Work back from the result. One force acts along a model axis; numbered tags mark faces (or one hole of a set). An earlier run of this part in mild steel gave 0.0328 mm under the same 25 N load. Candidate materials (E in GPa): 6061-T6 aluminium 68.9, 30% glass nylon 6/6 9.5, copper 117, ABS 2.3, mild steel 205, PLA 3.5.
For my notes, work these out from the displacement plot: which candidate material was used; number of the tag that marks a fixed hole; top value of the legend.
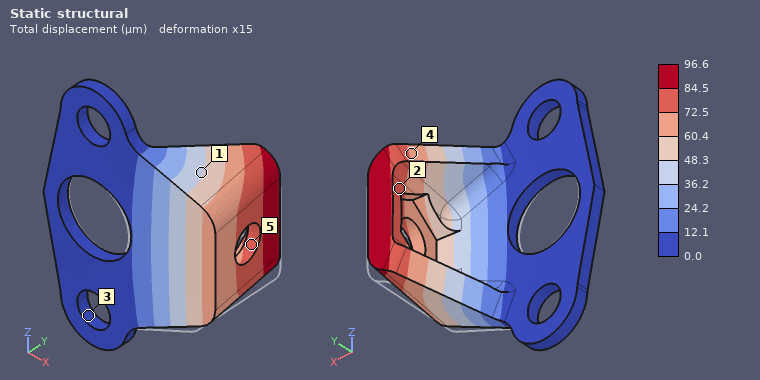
6061-T6 aluminium
3
96.6 µm
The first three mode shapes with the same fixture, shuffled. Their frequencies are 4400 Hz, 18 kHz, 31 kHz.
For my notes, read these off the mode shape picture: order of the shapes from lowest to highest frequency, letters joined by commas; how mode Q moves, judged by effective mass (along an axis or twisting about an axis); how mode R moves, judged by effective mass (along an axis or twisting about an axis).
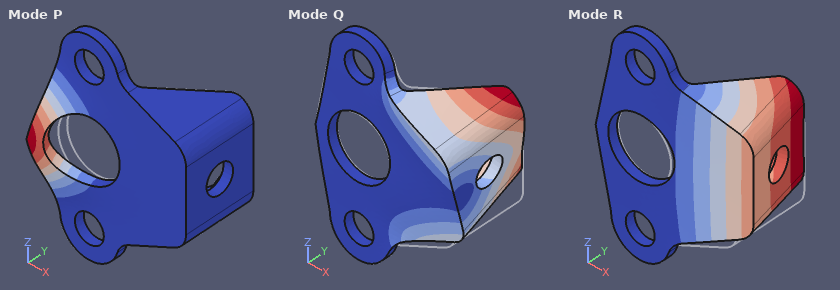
R, Q, P
along Z
along Y
